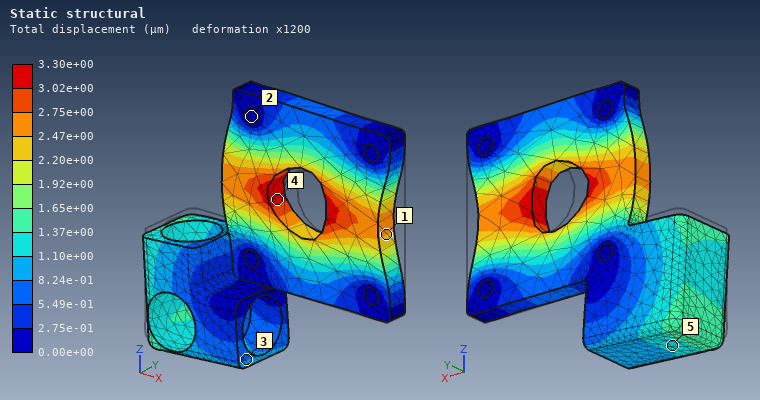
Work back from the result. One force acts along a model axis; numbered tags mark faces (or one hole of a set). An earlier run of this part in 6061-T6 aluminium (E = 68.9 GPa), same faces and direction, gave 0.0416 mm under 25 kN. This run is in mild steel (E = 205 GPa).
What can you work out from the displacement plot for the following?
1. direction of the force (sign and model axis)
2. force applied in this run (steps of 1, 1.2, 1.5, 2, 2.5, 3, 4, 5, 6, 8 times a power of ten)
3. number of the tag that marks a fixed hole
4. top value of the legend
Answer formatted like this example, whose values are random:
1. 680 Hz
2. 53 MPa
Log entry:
1. -X
2. 6 kN
3. 2
4. 3.30e+00 µm
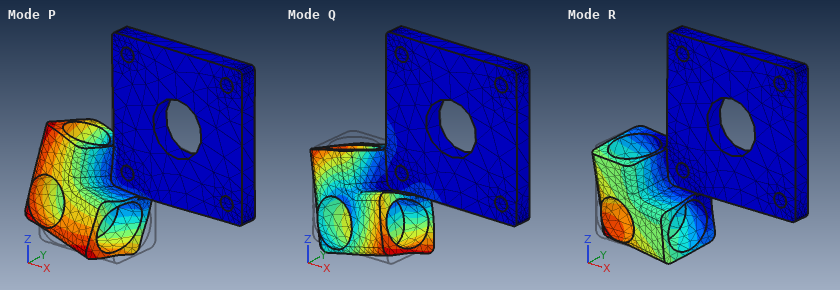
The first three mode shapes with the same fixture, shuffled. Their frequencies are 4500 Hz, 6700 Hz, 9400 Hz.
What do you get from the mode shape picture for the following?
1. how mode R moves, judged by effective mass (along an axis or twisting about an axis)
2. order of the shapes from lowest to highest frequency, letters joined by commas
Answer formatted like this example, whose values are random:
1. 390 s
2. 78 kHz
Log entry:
1. along Y
2. R, P, Q
